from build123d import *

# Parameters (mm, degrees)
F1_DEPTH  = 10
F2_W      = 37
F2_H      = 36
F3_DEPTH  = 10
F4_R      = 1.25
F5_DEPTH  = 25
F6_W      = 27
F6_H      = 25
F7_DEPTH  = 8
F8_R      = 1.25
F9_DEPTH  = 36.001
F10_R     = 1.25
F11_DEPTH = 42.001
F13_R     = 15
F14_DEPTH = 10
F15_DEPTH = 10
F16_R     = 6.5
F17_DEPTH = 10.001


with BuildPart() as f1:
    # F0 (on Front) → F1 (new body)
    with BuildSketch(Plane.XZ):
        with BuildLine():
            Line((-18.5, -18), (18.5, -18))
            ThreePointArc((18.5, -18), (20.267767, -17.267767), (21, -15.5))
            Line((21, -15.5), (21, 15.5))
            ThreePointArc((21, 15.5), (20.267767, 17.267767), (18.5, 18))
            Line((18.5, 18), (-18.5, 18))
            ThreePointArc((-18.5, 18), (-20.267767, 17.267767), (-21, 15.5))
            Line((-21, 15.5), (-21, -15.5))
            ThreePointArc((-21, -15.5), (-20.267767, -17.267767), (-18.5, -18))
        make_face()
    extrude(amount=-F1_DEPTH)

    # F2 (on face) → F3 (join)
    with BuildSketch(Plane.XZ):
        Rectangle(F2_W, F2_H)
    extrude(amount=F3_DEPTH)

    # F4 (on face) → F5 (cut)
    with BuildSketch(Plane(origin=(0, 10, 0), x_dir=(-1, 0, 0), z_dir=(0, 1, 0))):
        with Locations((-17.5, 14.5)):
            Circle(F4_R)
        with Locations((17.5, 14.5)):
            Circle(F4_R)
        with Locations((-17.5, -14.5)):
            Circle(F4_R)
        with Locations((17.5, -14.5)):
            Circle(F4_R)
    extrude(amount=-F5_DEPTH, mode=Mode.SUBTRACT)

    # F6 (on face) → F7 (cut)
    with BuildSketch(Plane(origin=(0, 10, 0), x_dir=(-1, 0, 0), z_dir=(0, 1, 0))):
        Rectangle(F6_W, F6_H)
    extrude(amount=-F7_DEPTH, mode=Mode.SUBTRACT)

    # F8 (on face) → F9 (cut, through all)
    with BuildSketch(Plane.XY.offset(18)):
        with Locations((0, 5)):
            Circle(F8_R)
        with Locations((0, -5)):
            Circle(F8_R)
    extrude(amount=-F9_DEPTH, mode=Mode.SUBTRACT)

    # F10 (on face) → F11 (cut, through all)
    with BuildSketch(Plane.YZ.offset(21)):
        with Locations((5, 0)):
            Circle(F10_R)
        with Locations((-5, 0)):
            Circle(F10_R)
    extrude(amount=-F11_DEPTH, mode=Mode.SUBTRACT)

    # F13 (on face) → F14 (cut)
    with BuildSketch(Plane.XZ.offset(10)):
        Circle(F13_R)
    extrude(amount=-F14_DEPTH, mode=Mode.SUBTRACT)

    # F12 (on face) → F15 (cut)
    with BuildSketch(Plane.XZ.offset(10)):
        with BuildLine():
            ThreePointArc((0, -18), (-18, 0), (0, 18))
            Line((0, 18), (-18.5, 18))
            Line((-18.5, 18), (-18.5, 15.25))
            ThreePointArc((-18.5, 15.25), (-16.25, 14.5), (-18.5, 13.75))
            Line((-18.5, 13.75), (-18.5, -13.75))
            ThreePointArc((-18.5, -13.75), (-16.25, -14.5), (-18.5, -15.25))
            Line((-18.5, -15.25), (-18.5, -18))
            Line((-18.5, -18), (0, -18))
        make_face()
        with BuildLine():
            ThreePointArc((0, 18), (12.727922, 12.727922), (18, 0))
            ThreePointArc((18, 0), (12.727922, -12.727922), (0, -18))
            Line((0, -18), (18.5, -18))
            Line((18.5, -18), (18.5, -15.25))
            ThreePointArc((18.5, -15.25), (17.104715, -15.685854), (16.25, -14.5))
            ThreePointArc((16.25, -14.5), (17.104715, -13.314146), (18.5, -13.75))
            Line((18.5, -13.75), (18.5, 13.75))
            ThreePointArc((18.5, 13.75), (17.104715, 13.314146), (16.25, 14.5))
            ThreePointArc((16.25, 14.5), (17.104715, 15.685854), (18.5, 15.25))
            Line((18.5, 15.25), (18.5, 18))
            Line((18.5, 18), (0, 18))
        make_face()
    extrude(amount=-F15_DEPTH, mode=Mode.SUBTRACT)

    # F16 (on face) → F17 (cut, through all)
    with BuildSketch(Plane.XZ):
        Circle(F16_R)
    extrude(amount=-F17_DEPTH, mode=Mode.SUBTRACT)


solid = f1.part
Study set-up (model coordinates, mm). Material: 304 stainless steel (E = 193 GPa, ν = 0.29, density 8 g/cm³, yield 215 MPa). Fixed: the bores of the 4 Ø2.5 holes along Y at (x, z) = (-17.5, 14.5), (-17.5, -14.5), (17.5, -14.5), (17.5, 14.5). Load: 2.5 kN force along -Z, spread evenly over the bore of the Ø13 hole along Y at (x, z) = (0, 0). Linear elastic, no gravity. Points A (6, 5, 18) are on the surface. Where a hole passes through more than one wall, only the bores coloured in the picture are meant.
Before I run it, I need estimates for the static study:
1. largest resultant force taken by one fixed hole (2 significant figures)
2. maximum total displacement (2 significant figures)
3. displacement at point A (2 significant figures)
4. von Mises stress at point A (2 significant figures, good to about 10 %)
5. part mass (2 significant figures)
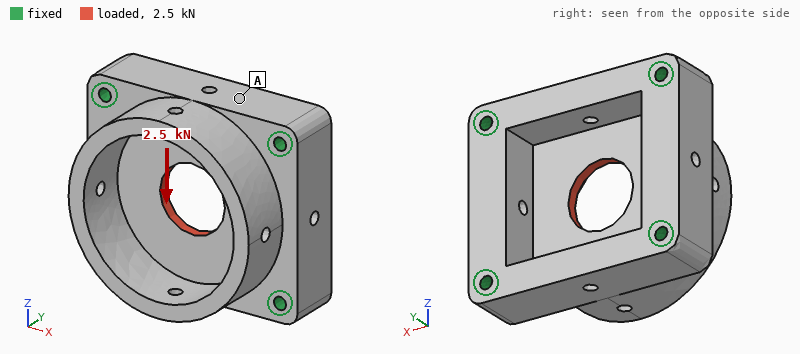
690 N
3.1 µm
1.5 µm
6.6 MPa
97 g
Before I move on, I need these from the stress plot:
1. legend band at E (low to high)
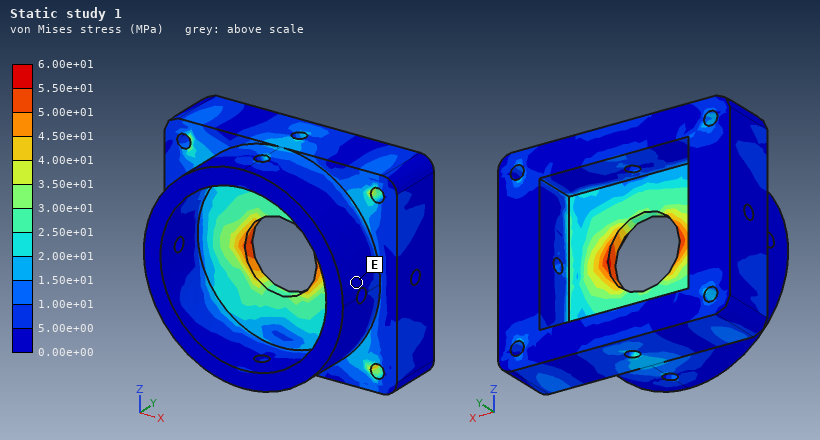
0.00e+00 to 5.00e+00 MPa
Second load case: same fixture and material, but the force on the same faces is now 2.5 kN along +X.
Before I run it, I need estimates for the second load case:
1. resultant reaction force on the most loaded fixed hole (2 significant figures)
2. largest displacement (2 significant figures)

670 N
2.4 µm
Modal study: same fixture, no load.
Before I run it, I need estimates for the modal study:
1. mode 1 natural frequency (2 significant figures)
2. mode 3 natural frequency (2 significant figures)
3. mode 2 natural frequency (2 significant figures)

20 kHz
25 kHz
24 kHz
